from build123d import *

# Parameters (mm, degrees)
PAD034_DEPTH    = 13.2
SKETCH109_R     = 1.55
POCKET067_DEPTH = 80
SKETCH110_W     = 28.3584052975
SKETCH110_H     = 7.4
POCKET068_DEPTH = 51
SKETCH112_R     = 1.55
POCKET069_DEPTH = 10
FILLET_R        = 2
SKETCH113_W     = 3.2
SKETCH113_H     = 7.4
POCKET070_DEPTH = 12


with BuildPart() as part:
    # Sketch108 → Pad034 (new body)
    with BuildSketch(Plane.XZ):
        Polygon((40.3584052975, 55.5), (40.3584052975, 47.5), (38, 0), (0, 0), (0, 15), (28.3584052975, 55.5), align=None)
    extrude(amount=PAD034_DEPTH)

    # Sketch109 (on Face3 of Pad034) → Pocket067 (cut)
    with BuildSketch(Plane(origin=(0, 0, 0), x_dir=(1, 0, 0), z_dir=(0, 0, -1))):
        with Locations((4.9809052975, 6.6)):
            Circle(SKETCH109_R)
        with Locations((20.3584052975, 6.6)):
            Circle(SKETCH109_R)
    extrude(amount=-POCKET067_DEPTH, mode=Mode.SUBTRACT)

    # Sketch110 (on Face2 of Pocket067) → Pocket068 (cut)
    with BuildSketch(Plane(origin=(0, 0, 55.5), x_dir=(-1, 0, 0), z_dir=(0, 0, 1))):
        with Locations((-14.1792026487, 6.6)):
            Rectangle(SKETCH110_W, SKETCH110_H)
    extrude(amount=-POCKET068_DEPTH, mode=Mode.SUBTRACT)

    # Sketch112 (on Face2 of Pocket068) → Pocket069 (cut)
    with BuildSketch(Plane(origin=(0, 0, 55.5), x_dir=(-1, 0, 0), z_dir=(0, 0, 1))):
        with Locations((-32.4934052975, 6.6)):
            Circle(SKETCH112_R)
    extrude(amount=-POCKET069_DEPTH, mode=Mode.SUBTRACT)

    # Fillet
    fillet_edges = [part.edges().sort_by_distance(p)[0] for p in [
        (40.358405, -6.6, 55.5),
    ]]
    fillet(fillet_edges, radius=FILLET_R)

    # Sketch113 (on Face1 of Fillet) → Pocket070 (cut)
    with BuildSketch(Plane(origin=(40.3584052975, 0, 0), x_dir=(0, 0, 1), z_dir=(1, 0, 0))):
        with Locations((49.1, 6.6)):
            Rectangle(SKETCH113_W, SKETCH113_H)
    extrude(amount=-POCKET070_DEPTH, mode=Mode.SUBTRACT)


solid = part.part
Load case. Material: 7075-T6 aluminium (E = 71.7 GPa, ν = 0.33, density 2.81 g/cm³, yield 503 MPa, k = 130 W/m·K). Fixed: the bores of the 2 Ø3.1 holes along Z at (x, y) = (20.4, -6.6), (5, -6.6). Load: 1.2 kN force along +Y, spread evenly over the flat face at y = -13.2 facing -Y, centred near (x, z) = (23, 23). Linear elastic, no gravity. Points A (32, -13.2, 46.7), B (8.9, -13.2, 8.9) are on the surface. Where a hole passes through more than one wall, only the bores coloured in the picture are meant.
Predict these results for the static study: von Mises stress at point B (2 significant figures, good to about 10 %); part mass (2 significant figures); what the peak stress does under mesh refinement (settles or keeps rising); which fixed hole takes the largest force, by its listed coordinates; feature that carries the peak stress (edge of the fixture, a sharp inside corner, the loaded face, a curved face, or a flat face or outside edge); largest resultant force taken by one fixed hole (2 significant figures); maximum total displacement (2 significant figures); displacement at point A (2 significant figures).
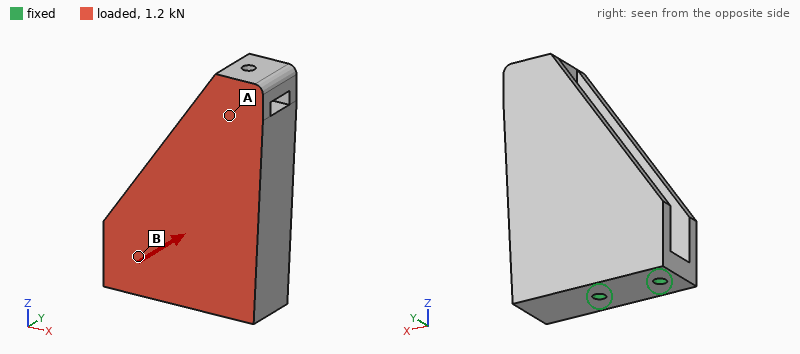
64 MPa
40 g
keeps rising
(20.4, -6.6)
edge of the fixture
1.3 kN
0.36 mm
0.29 mm
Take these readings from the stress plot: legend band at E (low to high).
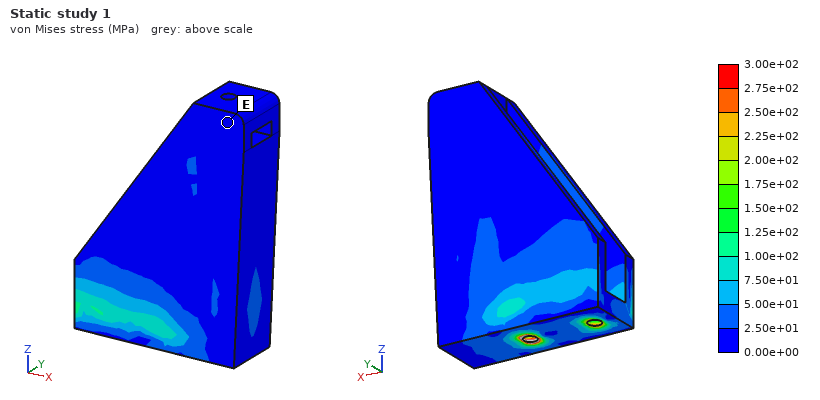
0.00e+00 to 2.50e+01 MPa
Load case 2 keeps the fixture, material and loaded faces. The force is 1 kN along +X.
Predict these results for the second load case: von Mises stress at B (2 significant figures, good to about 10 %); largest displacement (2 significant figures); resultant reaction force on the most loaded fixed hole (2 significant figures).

22 MPa
64 µm
1.3 kN
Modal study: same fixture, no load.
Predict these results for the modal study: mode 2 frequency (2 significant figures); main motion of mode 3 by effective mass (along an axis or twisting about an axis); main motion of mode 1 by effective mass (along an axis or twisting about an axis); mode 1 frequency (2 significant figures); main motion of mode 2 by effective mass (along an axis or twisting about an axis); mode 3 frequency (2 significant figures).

4000 Hz
twisting about Z
along Y
1900 Hz
along X
7300 Hz
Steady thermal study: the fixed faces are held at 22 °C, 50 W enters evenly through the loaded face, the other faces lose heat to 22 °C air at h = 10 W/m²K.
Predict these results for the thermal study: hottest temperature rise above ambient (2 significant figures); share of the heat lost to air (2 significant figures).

47 K
3.4 %
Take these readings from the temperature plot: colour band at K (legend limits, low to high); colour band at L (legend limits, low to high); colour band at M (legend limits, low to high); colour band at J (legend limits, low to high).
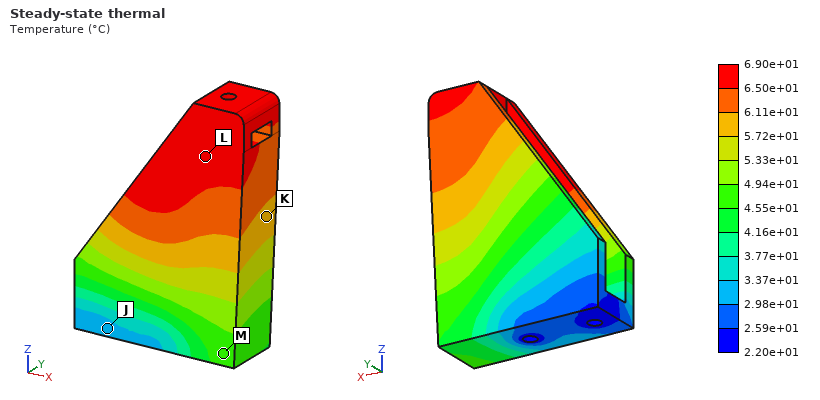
5.72e+01 to 6.11e+01 °C
6.50e+01 to 6.90e+01 °C
4.55e+01 to 4.94e+01 °C
2.98e+01 to 3.37e+01 °C
